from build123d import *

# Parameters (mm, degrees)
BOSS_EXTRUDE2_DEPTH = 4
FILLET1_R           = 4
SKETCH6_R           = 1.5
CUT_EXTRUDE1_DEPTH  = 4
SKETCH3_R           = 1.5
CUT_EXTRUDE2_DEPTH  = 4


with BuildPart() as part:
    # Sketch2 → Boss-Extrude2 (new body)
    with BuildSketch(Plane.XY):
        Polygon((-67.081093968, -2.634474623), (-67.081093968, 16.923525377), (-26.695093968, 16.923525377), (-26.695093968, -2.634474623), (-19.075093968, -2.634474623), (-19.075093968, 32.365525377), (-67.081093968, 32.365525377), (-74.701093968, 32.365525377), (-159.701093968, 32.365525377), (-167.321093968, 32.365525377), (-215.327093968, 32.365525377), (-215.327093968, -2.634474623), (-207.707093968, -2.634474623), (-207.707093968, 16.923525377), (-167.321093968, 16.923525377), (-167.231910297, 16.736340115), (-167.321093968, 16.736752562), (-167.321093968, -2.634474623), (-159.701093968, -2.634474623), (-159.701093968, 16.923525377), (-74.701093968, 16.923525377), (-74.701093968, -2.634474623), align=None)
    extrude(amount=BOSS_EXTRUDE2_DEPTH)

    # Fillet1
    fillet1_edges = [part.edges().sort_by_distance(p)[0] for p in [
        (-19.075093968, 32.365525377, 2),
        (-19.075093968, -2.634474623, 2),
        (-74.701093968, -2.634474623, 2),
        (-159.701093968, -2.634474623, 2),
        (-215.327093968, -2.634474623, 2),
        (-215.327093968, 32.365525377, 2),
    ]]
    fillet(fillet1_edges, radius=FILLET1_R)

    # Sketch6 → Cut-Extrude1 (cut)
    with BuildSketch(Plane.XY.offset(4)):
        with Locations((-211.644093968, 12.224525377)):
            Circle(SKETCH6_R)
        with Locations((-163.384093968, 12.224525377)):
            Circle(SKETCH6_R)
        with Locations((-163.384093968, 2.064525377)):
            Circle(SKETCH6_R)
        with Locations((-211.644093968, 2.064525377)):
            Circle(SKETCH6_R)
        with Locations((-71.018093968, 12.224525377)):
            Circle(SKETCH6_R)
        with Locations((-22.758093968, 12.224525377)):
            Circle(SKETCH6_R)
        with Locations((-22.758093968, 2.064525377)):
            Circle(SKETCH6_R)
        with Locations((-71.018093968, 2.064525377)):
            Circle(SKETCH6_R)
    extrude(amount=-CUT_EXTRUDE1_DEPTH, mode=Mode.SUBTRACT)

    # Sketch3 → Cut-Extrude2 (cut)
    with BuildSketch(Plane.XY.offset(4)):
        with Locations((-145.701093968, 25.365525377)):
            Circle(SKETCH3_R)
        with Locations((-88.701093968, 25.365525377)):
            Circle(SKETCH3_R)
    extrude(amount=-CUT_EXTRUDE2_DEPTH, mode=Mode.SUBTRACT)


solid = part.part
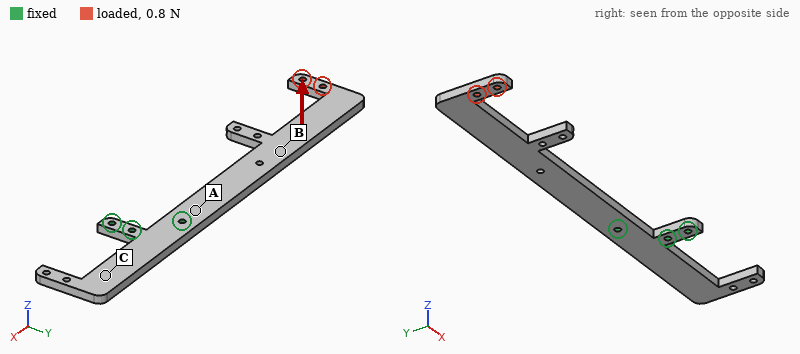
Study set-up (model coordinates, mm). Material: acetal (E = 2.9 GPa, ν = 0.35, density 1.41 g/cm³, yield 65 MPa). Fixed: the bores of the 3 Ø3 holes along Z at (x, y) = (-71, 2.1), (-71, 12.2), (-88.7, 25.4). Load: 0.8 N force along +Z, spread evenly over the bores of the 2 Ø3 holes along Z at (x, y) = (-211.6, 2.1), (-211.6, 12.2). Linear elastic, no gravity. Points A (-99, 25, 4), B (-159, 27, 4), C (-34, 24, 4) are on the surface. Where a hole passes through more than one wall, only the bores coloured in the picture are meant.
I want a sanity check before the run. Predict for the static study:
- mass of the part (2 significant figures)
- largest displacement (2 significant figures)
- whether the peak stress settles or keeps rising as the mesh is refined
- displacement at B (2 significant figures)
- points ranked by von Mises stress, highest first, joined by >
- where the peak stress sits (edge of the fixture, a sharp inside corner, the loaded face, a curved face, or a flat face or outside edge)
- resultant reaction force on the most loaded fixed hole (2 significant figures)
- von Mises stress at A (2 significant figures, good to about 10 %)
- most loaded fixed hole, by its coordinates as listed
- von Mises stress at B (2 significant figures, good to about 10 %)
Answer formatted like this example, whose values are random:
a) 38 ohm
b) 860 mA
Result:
a) 20 g
b) 2.3 mm
c) keeps rising
d) 0.81 mm
e) A > B > C
f) edge of the fixture
g) 1.6 N
h) 2.1 MPa
i) (-88.7, 25.4)
j) 1.1 MPa
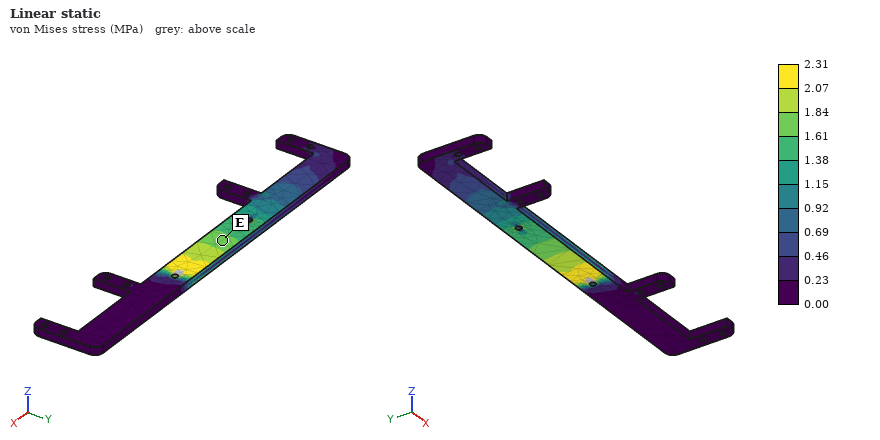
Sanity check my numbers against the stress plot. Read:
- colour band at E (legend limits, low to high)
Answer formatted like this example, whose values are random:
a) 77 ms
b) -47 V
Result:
a) 1.61 to 1.84 MPa
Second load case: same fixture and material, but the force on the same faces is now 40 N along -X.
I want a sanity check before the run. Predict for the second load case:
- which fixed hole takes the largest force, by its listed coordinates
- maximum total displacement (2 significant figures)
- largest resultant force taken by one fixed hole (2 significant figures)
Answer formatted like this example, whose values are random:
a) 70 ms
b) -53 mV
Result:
a) (-88.7, 25.4)
b) 2.0 mm
c) 43 N
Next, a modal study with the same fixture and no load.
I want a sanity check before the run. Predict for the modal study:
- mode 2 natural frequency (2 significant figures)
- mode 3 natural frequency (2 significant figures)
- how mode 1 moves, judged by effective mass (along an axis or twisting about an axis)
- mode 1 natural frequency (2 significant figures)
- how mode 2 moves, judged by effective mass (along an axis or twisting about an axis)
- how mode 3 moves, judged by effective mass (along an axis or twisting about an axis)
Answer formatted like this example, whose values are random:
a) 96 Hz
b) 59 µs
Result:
a) 170 Hz
b) 240 Hz
c) along Z
d) 51 Hz
e) along Y
f) along Z
